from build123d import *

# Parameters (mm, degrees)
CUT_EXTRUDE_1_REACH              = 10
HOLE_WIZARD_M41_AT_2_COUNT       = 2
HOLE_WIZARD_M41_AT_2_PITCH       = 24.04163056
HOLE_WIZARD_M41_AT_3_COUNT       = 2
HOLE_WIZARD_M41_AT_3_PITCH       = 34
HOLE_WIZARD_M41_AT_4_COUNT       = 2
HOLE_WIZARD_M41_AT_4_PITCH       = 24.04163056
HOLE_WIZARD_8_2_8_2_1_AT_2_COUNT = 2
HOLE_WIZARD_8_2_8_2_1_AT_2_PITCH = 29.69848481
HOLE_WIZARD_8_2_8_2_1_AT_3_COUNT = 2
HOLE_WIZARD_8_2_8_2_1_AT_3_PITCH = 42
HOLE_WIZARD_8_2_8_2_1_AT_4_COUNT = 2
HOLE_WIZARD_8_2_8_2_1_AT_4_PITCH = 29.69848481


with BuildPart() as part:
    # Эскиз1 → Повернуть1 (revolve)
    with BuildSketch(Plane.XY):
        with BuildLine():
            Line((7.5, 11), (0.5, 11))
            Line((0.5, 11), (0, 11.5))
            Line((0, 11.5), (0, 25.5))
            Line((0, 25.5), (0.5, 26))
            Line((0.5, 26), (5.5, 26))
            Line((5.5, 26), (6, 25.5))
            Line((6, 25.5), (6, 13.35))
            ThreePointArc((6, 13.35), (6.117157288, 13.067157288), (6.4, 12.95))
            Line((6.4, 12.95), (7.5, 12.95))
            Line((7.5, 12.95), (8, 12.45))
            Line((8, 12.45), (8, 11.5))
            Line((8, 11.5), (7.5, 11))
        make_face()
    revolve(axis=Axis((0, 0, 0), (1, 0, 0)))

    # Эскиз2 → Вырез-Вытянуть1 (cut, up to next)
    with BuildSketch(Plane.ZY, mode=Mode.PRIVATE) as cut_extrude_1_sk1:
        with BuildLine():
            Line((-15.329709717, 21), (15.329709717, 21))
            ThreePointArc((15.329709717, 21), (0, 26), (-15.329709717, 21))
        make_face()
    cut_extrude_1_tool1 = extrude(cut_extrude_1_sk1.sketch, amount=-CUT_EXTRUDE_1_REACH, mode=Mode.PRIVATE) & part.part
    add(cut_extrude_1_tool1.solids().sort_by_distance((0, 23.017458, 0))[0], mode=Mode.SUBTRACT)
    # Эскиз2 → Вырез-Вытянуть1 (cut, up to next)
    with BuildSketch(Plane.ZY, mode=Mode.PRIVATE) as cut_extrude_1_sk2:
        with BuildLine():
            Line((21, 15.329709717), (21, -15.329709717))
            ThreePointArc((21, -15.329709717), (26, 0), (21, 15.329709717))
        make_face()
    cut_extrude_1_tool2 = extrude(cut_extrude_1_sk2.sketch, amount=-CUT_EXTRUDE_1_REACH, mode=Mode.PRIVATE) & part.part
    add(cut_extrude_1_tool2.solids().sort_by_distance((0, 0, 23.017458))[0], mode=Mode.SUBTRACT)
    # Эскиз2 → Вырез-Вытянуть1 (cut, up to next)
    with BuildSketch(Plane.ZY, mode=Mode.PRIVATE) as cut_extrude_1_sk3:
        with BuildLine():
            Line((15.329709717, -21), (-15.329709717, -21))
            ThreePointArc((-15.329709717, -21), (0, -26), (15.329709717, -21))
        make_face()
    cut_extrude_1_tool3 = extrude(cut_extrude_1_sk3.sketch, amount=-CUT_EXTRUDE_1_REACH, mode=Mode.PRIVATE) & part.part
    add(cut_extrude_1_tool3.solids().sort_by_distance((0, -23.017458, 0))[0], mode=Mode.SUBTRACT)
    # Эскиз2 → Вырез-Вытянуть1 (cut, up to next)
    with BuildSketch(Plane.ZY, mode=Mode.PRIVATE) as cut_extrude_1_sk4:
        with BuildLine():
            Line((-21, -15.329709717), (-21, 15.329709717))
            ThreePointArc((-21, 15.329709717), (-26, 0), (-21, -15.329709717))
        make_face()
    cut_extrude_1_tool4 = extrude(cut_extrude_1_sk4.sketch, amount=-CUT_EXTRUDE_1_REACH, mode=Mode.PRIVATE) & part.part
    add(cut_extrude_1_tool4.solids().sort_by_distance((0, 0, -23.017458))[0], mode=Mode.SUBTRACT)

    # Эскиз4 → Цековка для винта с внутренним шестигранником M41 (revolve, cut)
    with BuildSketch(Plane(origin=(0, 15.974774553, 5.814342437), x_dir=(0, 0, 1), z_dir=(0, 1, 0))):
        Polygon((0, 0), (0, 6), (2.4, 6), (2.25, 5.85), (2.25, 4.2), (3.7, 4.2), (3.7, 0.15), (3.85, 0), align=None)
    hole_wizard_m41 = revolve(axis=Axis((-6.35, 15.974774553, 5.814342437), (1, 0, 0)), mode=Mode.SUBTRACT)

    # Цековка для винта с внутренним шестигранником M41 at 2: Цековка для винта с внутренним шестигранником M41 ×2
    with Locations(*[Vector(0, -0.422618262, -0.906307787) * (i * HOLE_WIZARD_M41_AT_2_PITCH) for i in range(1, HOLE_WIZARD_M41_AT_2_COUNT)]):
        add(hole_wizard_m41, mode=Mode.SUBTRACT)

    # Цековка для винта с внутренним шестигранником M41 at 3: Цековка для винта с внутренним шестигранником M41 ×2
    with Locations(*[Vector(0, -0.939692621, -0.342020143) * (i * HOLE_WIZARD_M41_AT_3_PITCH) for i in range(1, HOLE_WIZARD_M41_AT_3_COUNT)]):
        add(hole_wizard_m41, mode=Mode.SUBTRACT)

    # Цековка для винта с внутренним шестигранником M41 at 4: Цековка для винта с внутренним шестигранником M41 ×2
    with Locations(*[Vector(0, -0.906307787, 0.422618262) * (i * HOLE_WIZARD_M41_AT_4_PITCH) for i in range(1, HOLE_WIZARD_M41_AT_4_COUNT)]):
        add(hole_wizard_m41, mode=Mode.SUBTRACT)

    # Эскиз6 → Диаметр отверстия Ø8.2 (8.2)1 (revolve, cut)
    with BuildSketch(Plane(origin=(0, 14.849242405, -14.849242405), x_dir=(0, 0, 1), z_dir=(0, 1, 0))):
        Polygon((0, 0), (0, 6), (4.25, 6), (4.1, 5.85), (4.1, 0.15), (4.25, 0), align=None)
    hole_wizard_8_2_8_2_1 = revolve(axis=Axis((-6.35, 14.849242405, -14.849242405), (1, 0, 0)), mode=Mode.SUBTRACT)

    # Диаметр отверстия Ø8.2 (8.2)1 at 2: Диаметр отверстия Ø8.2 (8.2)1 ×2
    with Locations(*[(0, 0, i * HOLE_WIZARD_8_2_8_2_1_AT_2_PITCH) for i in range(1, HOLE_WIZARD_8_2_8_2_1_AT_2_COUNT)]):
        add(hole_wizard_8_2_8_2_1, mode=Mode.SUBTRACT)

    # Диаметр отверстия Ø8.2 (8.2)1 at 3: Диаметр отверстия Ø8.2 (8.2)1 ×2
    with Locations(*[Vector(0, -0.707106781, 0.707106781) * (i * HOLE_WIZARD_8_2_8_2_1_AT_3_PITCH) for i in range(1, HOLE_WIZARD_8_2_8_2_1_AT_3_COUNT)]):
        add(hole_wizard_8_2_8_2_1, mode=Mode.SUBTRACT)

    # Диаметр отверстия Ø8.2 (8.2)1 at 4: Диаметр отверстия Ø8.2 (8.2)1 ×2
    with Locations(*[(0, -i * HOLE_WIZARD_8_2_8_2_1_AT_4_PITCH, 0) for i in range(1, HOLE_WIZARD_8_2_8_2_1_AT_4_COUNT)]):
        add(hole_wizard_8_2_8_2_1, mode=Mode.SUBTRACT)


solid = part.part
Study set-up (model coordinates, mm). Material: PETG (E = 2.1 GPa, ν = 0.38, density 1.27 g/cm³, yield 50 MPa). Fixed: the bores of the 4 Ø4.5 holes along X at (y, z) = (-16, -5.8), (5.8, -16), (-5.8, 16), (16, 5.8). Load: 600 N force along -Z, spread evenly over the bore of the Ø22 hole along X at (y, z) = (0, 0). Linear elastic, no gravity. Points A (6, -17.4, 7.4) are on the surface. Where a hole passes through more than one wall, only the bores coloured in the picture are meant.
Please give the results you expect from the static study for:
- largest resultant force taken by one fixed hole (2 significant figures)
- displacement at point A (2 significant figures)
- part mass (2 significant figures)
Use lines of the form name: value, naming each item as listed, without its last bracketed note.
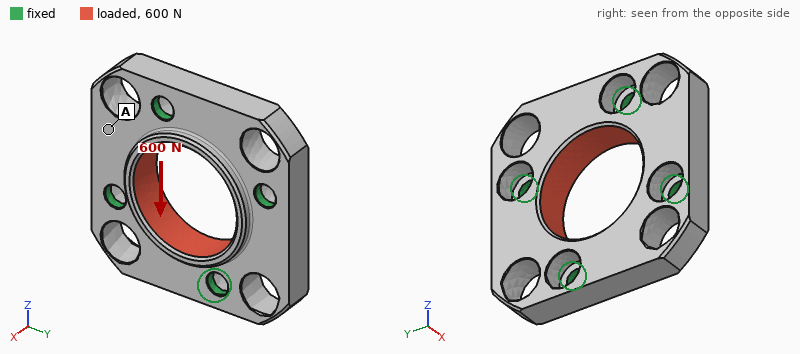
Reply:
largest resultant force taken by one fixed hole: 150 N
displacement at point A: 15 µm
part mass: 7.8 g
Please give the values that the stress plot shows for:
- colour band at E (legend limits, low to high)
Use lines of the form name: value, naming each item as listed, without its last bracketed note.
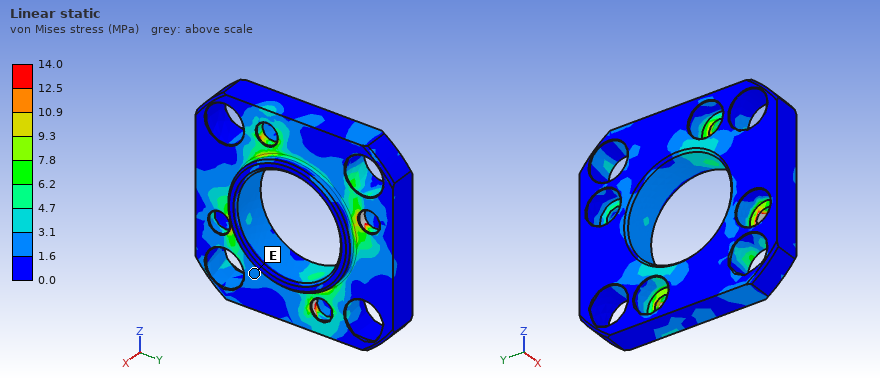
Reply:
colour band at E: 1.6 to 3.1 MPa
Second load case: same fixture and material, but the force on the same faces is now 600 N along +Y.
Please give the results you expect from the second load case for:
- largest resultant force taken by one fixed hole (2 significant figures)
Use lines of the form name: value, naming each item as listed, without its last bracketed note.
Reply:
largest resultant force taken by one fixed hole: 150 N
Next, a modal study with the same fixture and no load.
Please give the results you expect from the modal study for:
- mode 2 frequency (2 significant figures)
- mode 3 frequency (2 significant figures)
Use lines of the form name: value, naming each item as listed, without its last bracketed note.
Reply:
mode 2 frequency: 4600 Hz
mode 3 frequency: 4600 Hz
